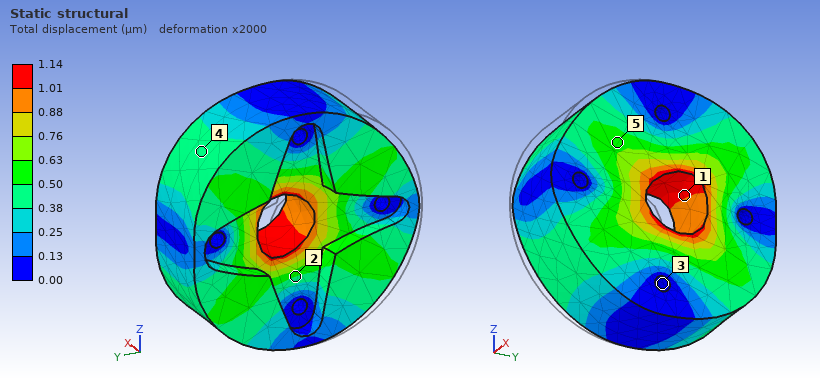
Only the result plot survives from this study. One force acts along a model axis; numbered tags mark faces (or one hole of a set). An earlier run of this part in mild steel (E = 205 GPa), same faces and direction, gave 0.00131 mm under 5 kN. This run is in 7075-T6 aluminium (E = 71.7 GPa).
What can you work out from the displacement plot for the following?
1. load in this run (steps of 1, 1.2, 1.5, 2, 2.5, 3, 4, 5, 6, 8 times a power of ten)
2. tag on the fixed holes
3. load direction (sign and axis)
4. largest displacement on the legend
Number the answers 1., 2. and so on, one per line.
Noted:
1. 1.5 kN
2. 3
3. +Y
4. 1.14 µm
